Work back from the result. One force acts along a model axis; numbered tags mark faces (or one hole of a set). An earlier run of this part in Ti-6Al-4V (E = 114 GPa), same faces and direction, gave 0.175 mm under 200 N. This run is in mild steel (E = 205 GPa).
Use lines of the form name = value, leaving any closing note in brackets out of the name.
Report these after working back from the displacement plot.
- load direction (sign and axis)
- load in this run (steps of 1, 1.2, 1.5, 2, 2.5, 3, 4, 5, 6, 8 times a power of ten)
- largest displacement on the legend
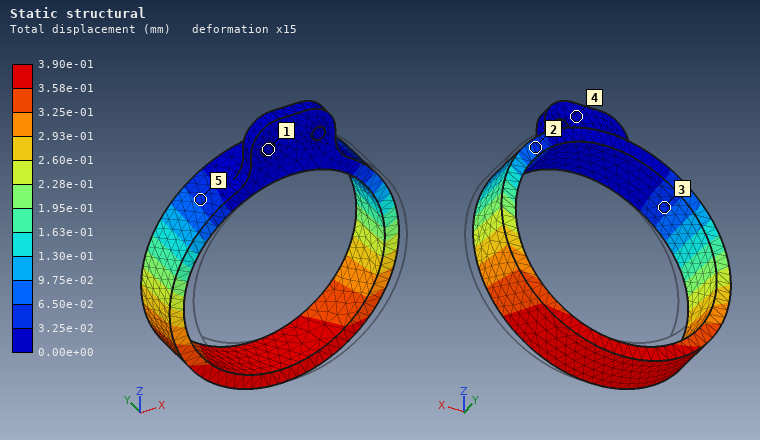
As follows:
load direction = -X
load in this run = 800 N
largest displacement on the legend = 3.90e-01 mm
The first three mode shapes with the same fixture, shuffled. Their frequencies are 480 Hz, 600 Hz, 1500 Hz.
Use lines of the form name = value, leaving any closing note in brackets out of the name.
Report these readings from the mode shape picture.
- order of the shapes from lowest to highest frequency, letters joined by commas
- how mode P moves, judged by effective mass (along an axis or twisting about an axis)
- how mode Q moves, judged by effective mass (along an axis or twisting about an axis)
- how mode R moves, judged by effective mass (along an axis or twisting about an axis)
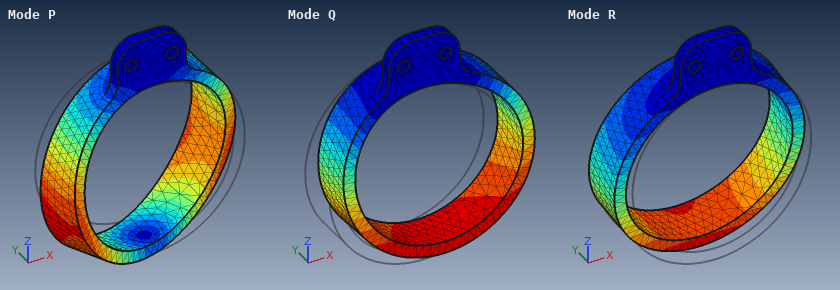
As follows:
order of the shapes from lowest to highest frequency, letters joined by commas = R, Q, P
how mode P moves, judged by effective mass = twisting about Z
how mode Q moves, judged by effective mass = along X
how mode R moves, judged by effective mass = along Y
